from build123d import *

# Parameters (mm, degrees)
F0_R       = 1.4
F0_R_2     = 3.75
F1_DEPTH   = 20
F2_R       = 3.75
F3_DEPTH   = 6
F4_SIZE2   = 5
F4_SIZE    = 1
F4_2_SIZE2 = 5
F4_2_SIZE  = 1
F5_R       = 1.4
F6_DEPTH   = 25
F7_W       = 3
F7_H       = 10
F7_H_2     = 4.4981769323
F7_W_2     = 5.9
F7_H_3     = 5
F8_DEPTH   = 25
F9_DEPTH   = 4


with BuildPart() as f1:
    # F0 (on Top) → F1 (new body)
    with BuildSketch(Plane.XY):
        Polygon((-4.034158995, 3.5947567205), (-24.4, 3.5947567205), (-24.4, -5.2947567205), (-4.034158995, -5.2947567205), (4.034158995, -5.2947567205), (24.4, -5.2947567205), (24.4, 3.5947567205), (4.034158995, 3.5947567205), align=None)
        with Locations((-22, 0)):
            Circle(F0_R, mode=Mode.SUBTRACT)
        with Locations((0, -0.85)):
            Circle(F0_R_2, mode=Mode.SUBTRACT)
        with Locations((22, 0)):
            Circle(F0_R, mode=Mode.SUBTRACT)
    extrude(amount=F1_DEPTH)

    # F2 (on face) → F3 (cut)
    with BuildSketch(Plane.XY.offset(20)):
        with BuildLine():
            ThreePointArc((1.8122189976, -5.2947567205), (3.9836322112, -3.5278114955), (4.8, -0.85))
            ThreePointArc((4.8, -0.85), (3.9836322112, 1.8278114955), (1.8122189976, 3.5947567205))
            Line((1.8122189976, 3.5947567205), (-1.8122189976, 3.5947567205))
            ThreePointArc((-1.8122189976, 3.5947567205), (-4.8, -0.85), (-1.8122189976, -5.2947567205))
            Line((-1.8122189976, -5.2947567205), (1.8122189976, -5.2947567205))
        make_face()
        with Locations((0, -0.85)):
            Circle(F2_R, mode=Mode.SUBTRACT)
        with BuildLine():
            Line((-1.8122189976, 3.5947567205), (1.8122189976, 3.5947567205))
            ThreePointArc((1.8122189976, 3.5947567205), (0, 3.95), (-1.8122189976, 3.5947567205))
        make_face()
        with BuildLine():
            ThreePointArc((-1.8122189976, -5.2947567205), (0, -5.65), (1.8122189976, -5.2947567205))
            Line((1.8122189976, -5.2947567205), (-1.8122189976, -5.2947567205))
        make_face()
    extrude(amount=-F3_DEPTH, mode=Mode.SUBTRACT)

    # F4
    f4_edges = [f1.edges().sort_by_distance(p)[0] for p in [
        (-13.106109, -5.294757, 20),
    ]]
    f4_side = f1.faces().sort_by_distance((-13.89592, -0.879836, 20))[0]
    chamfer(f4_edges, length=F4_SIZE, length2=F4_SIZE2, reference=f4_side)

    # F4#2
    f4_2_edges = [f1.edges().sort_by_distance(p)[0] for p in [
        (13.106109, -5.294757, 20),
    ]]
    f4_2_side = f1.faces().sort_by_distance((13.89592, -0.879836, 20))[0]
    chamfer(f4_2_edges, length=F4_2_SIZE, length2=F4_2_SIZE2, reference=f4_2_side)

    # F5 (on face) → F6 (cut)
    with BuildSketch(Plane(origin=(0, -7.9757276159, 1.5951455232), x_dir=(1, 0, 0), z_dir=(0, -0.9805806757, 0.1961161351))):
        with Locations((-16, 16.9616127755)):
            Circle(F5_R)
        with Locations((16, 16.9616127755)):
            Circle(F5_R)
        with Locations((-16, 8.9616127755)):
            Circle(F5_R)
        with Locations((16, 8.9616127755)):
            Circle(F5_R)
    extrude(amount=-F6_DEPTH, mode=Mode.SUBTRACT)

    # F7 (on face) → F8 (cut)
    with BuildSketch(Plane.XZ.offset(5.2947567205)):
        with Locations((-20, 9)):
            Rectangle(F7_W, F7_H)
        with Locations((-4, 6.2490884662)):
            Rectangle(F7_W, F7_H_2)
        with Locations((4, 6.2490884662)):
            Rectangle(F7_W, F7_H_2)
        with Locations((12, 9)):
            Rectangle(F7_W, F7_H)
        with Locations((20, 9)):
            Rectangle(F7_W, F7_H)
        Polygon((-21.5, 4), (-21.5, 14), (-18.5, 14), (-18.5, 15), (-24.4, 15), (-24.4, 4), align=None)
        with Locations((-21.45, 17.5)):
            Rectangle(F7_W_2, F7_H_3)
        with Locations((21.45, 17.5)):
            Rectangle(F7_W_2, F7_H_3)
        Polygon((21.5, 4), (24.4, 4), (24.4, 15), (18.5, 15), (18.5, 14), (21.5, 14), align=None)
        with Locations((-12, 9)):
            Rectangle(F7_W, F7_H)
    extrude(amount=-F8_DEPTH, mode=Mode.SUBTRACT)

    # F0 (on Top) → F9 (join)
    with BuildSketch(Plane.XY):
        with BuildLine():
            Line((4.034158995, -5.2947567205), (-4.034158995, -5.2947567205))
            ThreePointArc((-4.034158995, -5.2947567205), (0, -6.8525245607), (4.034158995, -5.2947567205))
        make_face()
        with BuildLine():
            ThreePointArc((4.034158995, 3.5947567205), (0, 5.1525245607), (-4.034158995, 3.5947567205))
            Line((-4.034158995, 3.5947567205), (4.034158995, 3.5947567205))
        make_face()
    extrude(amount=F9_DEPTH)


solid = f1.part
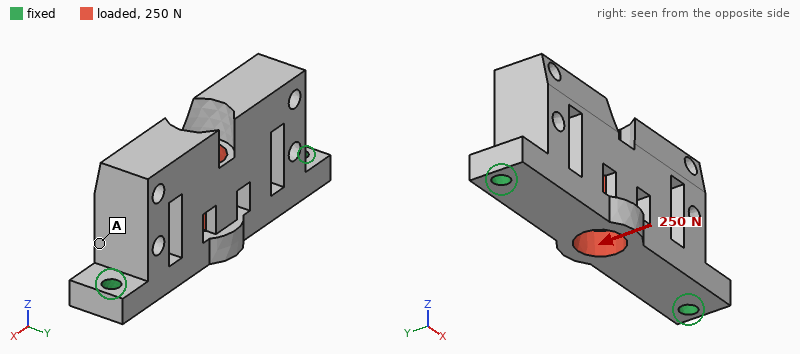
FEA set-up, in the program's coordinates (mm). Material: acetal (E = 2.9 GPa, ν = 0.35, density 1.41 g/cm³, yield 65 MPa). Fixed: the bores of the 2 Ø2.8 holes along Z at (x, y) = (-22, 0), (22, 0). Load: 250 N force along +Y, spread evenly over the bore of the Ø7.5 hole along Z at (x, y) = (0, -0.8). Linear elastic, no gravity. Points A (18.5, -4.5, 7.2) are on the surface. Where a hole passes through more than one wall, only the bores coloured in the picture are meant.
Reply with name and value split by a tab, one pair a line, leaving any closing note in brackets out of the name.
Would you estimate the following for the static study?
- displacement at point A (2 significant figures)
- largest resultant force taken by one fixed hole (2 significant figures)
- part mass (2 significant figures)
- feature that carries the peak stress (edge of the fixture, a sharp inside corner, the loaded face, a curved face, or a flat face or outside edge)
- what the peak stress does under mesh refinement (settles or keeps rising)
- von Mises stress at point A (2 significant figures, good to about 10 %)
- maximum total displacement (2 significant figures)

displacement at point A	0.15 mm
largest resultant force taken by one fixed hole	130 N
part mass	7.0 g
feature that carries the peak stress	edge of the fixture
what the peak stress does under mesh refinement	keeps rising
von Mises stress at point A	7.4 MPa
maximum total displacement	0.57 mm
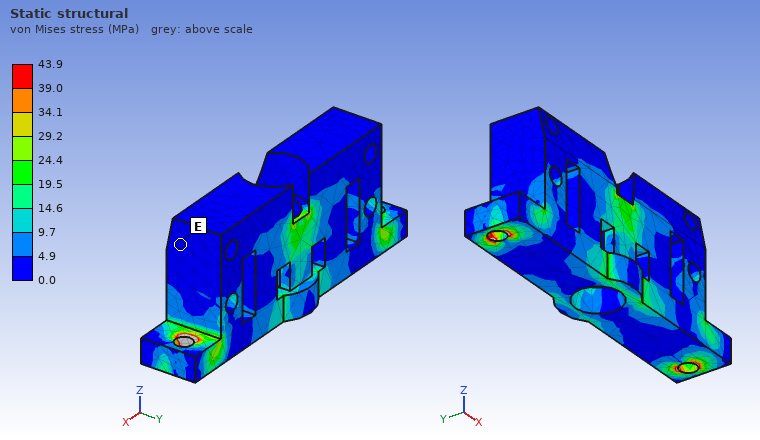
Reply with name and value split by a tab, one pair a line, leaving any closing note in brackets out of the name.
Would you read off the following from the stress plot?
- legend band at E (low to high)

legend band at E	0.0 to 4.9 MPa
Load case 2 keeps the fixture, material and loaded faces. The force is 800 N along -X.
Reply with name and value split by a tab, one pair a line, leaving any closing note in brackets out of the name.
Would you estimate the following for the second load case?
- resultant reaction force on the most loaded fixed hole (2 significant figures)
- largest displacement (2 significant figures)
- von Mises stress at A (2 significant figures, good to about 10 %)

resultant reaction force on the most loaded fixed hole	410 N
largest displacement	0.14 mm
von Mises stress at A	8.5 MPa
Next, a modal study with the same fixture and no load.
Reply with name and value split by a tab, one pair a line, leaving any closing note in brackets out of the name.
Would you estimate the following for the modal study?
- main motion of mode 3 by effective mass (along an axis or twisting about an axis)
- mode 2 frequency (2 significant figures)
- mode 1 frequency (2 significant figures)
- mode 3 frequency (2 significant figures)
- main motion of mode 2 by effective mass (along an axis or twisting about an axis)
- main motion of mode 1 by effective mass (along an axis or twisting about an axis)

main motion of mode 3 by effective mass	along Z
mode 2 frequency	3000 Hz
mode 1 frequency	1500 Hz
mode 3 frequency	3200 Hz
main motion of mode 2 by effective mass	twisting about Z
main motion of mode 1 by effective mass	along Y
